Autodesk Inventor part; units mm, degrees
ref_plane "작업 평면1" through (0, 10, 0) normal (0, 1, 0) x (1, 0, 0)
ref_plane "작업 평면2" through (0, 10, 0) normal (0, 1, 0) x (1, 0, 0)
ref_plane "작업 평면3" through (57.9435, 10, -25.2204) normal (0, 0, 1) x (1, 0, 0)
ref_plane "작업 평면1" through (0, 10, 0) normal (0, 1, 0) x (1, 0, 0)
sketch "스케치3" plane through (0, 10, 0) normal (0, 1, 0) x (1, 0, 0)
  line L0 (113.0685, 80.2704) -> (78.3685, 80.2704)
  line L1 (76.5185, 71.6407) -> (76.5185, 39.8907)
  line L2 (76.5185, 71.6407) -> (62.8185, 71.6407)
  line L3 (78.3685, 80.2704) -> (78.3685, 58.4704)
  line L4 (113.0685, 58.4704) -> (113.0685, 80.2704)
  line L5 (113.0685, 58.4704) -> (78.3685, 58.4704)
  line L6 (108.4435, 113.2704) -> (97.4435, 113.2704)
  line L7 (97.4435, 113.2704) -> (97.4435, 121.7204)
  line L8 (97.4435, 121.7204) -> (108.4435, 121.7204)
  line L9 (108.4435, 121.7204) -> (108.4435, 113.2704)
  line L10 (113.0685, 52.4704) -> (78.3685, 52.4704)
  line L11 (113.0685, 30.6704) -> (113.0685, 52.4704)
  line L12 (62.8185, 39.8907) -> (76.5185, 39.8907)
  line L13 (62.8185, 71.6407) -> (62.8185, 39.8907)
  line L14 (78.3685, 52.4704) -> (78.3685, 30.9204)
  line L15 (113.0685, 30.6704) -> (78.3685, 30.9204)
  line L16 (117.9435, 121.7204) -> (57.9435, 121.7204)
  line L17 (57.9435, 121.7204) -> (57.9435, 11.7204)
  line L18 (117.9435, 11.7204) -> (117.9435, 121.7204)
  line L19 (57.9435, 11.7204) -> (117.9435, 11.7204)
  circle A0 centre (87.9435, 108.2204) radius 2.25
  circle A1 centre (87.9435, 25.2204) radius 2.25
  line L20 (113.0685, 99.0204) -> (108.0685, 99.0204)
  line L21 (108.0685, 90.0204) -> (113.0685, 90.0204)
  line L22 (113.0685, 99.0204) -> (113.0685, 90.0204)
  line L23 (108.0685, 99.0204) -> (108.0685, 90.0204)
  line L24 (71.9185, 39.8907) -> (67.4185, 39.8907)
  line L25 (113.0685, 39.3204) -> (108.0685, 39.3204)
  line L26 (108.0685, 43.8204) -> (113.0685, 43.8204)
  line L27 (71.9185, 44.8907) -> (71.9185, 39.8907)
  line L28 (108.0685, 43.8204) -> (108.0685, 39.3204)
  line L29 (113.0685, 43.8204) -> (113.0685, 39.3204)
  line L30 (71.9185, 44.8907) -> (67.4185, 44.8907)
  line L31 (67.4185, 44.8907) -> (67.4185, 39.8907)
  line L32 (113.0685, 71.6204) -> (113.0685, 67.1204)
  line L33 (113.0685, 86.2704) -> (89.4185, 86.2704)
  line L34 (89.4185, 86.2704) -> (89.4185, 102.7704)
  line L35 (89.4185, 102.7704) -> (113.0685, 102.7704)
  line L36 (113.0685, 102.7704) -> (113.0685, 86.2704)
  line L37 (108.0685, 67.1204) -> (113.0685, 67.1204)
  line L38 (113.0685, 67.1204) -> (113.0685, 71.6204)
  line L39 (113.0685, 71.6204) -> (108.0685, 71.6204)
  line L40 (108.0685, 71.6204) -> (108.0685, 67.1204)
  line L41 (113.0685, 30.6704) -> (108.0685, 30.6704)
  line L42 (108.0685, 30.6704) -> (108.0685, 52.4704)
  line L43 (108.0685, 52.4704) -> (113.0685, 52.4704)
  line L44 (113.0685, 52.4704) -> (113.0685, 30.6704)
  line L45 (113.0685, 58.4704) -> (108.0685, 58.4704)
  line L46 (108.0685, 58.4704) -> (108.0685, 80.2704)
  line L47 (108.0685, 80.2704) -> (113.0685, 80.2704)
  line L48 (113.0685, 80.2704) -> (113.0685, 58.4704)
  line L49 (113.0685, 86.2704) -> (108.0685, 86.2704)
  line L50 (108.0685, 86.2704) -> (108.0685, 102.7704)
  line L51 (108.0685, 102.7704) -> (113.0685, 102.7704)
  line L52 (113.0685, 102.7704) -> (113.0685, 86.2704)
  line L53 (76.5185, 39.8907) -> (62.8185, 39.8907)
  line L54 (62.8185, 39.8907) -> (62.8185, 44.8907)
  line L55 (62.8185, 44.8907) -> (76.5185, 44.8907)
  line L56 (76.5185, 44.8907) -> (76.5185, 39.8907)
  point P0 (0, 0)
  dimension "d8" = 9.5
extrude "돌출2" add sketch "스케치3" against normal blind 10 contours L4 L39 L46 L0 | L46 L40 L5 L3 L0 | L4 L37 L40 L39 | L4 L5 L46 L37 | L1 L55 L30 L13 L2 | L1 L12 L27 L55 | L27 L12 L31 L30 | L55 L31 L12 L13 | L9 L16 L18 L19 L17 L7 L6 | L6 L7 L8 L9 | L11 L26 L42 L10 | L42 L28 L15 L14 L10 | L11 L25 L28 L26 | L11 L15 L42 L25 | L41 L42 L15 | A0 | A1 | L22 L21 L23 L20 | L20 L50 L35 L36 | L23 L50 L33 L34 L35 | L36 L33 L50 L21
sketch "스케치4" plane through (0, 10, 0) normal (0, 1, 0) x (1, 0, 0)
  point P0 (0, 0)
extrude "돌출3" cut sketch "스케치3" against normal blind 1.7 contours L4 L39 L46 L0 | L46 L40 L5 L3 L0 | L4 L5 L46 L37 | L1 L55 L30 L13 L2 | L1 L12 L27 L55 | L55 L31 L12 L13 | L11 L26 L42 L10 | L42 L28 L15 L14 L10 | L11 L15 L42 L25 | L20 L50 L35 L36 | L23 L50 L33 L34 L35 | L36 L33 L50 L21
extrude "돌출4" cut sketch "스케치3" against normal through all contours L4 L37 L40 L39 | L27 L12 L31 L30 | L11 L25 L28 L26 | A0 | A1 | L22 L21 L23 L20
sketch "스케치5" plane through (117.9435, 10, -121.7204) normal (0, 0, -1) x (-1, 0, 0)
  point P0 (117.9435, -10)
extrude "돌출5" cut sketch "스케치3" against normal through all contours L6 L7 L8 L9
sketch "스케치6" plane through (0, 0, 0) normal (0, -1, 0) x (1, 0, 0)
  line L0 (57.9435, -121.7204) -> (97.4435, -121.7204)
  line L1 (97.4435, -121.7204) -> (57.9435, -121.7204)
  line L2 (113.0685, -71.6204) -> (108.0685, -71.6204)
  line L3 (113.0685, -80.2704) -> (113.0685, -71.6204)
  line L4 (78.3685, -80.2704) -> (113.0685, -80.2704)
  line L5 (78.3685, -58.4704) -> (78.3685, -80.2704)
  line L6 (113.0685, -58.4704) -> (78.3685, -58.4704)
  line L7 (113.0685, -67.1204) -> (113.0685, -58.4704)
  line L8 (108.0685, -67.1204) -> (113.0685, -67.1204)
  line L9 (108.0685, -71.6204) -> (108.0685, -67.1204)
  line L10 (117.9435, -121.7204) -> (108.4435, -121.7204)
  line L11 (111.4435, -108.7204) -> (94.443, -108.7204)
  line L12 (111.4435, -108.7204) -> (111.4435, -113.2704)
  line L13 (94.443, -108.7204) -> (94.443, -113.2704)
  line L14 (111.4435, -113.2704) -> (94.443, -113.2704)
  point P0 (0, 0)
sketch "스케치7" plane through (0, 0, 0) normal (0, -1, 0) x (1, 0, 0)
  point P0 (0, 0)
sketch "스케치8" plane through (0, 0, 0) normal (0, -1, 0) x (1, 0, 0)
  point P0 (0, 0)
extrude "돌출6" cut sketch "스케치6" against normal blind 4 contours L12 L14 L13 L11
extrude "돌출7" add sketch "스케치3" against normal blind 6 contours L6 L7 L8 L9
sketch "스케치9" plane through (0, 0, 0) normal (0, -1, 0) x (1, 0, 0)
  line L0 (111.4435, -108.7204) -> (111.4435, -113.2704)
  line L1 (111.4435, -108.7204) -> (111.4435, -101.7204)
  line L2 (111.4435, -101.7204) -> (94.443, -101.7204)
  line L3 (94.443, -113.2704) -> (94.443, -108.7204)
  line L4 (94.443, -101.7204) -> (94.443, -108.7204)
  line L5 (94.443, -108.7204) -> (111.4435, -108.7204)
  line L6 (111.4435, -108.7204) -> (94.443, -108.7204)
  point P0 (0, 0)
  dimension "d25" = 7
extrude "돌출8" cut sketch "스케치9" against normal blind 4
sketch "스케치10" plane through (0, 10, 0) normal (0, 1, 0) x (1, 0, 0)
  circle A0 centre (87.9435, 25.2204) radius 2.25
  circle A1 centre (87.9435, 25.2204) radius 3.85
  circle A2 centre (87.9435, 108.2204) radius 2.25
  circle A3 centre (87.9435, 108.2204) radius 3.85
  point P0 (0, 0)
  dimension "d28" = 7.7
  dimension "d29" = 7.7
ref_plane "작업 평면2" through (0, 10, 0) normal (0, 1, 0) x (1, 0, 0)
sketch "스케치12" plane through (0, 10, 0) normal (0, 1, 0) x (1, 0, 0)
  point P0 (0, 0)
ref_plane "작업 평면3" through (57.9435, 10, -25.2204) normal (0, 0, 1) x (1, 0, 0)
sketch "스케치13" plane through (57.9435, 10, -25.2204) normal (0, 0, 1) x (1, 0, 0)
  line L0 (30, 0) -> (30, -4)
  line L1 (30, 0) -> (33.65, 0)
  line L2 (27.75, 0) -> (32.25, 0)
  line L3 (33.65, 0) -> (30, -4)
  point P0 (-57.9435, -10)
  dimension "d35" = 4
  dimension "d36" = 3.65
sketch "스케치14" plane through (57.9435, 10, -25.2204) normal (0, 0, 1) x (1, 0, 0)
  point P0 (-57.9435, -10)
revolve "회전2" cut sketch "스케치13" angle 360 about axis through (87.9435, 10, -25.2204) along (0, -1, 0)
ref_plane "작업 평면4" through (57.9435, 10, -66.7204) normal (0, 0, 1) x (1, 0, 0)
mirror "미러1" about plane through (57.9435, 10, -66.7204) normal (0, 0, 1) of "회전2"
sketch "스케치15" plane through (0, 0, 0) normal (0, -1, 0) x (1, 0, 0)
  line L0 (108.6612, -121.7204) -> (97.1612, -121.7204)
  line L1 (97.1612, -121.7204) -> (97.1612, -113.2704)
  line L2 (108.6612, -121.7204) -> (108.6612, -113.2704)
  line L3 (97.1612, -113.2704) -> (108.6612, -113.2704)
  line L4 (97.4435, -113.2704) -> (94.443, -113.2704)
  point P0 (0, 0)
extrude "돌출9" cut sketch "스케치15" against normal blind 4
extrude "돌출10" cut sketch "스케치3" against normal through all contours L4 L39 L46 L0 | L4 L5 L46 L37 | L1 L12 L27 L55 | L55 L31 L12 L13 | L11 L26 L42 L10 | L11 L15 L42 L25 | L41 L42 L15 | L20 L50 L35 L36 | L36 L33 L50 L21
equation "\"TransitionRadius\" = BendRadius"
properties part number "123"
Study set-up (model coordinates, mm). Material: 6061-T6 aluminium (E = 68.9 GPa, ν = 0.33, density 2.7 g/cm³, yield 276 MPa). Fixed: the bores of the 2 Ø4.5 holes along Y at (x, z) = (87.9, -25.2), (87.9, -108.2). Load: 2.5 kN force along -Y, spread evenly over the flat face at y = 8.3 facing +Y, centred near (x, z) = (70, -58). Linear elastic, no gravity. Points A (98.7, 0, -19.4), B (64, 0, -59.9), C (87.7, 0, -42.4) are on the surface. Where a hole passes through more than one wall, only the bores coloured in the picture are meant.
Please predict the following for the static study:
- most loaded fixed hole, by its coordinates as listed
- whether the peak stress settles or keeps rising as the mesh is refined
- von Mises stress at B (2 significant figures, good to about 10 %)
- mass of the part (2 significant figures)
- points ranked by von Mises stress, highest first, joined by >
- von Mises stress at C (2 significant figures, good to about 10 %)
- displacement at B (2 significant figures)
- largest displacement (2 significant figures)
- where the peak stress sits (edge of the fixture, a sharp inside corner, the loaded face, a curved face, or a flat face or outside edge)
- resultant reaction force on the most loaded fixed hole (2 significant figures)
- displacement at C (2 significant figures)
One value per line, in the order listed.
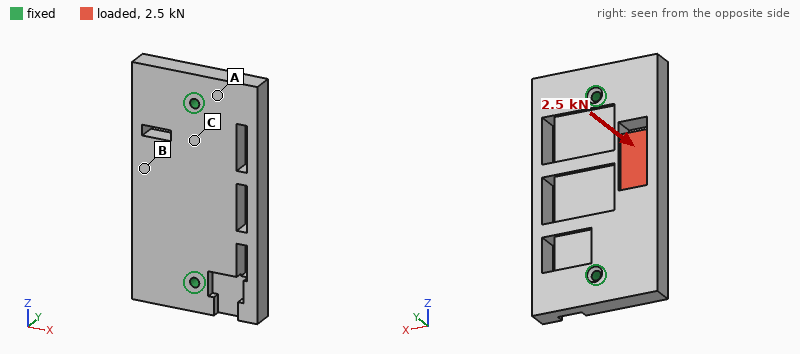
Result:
(87.9, -25.2)
keeps rising
45 MPa
160 g
B > C > A
28 MPa
0.12 mm
0.14 mm
edge of the fixture
1.6 kN
0.029 mm
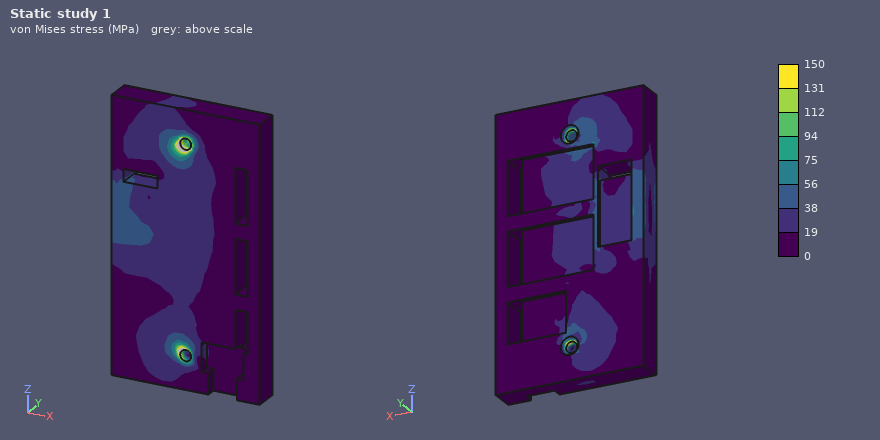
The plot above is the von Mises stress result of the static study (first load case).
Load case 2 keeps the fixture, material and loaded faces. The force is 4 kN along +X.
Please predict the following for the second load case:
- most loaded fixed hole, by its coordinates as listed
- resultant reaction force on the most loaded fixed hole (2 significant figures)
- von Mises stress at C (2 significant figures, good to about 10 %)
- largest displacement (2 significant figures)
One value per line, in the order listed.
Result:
(87.9, -25.2)
2.4 kN
11 MPa
45 µm
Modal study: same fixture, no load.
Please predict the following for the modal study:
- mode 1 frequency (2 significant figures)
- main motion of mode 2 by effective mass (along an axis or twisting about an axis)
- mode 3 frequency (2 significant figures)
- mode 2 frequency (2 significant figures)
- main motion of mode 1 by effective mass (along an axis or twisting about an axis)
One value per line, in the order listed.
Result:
3800 Hz
along Y
6400 Hz
4400 Hz
twisting about Z
